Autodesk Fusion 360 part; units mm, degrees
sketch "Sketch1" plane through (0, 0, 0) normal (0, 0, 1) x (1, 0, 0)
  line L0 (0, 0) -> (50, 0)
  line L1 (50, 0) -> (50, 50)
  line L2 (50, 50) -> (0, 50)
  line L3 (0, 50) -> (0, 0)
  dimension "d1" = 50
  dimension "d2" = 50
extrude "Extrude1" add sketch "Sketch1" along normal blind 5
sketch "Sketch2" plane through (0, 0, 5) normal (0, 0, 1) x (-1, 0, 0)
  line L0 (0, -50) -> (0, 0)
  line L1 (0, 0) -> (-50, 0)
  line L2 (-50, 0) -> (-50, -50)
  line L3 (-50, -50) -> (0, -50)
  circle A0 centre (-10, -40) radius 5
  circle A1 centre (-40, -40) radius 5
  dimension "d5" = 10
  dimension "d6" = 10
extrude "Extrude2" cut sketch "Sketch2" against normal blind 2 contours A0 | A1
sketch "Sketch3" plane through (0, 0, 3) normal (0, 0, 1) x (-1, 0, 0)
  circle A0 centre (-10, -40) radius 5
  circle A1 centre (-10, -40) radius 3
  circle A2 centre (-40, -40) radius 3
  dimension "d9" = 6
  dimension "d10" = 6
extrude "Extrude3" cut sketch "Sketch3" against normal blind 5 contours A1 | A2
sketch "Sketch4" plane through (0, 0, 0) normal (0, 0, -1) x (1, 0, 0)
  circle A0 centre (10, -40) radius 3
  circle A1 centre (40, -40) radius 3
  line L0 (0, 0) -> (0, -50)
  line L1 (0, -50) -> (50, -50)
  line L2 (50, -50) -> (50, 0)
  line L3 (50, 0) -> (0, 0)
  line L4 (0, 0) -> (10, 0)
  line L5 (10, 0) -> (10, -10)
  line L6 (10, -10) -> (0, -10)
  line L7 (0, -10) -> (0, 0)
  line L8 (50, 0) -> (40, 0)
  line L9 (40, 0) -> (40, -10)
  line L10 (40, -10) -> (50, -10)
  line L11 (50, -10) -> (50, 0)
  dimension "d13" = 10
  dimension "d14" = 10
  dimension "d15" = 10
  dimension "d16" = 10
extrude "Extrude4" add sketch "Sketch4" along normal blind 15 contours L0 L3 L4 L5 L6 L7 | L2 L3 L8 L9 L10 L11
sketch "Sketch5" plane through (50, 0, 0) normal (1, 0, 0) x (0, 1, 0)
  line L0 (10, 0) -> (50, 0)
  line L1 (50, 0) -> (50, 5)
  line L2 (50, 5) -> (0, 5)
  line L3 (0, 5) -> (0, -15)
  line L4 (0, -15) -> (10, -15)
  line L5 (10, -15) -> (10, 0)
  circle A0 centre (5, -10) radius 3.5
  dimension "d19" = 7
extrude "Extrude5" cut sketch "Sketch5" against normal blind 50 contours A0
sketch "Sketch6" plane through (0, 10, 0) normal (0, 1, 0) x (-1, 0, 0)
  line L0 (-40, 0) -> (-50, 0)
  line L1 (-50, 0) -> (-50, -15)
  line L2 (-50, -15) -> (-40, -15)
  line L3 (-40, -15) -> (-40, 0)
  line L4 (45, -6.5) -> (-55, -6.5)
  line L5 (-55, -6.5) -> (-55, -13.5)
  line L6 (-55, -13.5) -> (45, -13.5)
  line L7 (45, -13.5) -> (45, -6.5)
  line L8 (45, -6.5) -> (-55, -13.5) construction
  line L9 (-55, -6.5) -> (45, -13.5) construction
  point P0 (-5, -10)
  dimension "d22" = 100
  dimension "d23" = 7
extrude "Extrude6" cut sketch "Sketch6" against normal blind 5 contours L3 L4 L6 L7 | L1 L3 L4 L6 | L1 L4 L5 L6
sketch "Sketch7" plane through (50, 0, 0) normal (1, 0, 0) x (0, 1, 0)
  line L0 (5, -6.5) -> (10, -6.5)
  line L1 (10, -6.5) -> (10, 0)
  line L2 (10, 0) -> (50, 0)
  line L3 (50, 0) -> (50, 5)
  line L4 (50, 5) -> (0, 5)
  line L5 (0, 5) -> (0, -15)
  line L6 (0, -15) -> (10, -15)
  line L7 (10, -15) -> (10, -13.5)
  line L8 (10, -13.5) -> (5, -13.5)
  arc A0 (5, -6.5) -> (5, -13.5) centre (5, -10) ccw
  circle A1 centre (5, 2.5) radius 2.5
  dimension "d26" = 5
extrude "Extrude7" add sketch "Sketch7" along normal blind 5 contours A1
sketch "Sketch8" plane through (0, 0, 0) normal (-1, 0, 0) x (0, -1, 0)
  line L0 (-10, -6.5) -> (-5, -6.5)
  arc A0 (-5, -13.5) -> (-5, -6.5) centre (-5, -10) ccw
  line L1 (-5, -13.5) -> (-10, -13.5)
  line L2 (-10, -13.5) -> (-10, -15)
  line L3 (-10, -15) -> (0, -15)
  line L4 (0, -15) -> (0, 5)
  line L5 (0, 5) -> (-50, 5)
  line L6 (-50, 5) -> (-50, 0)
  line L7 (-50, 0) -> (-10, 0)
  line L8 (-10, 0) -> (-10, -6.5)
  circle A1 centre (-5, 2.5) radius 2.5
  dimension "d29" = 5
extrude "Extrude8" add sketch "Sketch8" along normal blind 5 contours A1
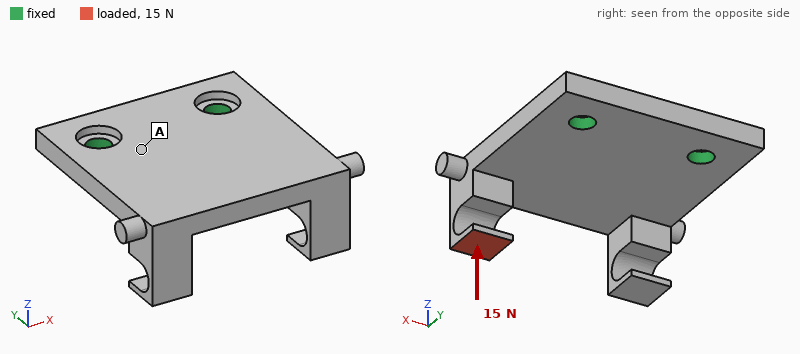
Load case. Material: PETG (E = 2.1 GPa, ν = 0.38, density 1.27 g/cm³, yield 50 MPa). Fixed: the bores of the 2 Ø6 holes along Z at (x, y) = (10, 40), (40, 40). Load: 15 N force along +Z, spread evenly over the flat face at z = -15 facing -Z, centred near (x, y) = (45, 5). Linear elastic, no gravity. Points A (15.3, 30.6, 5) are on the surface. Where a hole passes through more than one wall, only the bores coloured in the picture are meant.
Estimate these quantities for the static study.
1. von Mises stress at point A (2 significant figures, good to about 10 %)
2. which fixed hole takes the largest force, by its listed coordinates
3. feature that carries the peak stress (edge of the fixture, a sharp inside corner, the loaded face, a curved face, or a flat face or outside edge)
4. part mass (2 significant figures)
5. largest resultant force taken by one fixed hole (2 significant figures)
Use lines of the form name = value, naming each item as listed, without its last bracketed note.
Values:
von Mises stress at point A = 1.3 MPa
which fixed hole takes the largest force, by its listed coordinates = (40, 40)
feature that carries the peak stress = a curved face
part mass = 18 g
largest resultant force taken by one fixed hole = 17 N
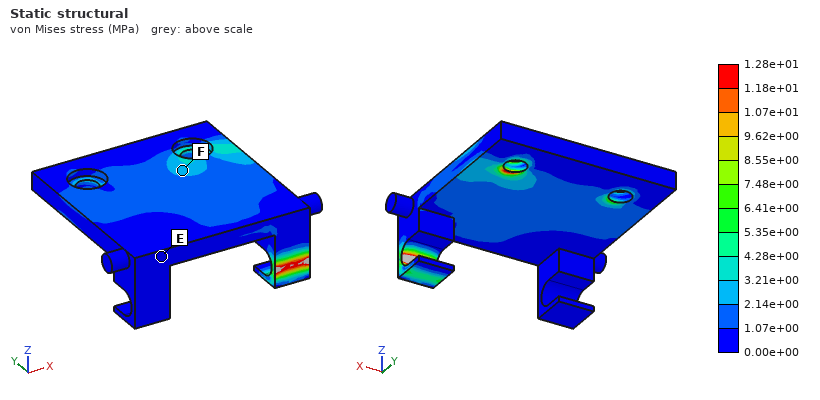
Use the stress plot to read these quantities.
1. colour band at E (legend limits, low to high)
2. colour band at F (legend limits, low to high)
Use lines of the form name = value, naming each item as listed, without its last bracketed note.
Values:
colour band at E = 0.00e+00 to 1.07e+00 MPa
colour band at F = 2.14e+00 to 3.21e+00 MPa
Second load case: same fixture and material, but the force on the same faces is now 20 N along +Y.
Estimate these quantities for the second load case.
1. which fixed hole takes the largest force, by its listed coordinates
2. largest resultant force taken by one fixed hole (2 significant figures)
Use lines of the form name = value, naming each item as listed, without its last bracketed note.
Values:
which fixed hole takes the largest force, by its listed coordinates = (40, 40)
largest resultant force taken by one fixed hole = 23 N
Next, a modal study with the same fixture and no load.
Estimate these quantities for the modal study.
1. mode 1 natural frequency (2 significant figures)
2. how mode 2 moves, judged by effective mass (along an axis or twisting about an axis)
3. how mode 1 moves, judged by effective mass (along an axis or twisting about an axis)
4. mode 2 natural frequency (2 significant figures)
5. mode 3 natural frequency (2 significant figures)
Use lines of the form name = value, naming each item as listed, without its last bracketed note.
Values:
mode 1 natural frequency = 430 Hz
how mode 2 moves, judged by effective mass = twisting about Y
how mode 1 moves, judged by effective mass = along Z
mode 2 natural frequency = 800 Hz
mode 3 natural frequency = 1800 Hz
